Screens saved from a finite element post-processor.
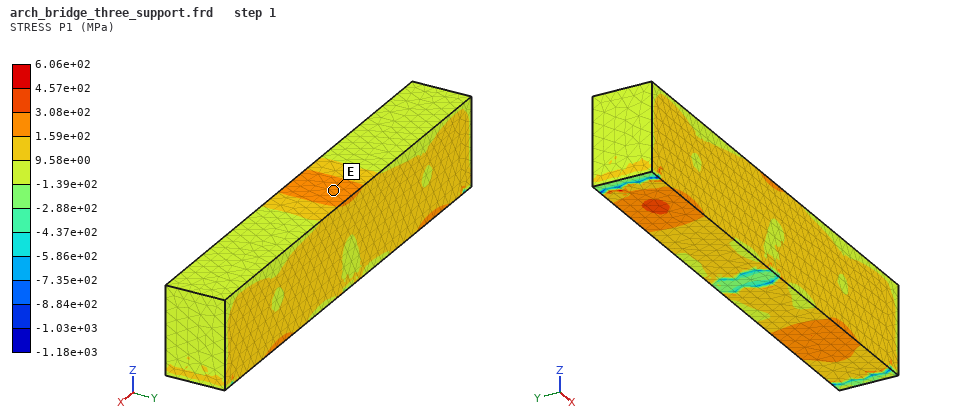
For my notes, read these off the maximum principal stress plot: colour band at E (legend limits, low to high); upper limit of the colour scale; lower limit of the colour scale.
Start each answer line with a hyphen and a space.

- 1.59e+02 to 3.08e+02 MPa
- 6.06e+02 MPa
- -1.18e+03 MPa
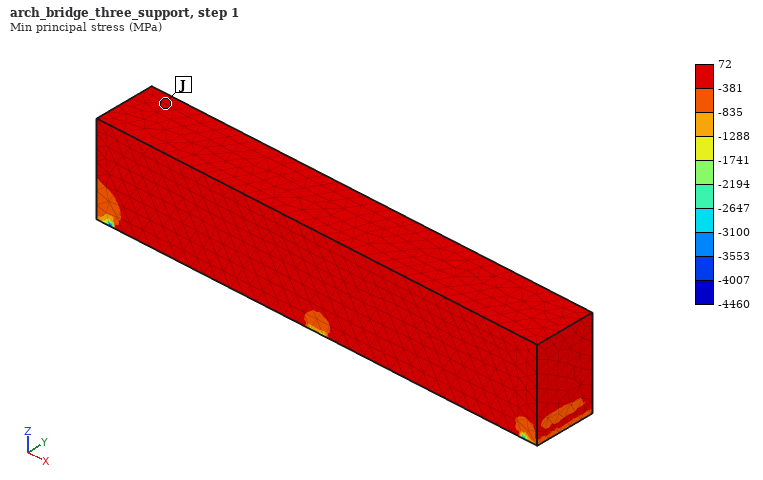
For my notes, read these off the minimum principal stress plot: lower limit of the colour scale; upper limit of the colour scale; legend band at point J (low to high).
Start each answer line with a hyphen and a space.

- -4460 MPa
- 72 MPa
- -381 to 72 MPa
